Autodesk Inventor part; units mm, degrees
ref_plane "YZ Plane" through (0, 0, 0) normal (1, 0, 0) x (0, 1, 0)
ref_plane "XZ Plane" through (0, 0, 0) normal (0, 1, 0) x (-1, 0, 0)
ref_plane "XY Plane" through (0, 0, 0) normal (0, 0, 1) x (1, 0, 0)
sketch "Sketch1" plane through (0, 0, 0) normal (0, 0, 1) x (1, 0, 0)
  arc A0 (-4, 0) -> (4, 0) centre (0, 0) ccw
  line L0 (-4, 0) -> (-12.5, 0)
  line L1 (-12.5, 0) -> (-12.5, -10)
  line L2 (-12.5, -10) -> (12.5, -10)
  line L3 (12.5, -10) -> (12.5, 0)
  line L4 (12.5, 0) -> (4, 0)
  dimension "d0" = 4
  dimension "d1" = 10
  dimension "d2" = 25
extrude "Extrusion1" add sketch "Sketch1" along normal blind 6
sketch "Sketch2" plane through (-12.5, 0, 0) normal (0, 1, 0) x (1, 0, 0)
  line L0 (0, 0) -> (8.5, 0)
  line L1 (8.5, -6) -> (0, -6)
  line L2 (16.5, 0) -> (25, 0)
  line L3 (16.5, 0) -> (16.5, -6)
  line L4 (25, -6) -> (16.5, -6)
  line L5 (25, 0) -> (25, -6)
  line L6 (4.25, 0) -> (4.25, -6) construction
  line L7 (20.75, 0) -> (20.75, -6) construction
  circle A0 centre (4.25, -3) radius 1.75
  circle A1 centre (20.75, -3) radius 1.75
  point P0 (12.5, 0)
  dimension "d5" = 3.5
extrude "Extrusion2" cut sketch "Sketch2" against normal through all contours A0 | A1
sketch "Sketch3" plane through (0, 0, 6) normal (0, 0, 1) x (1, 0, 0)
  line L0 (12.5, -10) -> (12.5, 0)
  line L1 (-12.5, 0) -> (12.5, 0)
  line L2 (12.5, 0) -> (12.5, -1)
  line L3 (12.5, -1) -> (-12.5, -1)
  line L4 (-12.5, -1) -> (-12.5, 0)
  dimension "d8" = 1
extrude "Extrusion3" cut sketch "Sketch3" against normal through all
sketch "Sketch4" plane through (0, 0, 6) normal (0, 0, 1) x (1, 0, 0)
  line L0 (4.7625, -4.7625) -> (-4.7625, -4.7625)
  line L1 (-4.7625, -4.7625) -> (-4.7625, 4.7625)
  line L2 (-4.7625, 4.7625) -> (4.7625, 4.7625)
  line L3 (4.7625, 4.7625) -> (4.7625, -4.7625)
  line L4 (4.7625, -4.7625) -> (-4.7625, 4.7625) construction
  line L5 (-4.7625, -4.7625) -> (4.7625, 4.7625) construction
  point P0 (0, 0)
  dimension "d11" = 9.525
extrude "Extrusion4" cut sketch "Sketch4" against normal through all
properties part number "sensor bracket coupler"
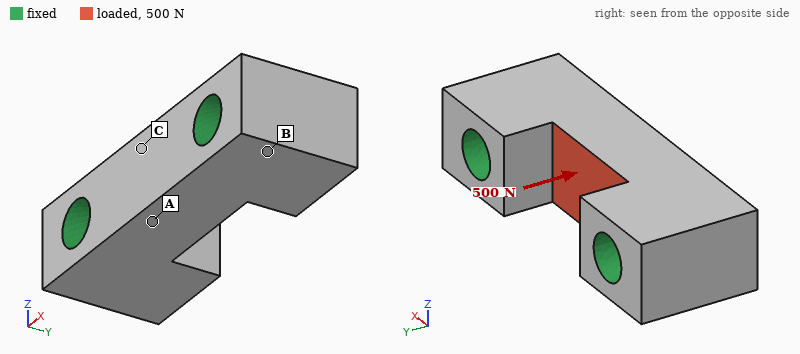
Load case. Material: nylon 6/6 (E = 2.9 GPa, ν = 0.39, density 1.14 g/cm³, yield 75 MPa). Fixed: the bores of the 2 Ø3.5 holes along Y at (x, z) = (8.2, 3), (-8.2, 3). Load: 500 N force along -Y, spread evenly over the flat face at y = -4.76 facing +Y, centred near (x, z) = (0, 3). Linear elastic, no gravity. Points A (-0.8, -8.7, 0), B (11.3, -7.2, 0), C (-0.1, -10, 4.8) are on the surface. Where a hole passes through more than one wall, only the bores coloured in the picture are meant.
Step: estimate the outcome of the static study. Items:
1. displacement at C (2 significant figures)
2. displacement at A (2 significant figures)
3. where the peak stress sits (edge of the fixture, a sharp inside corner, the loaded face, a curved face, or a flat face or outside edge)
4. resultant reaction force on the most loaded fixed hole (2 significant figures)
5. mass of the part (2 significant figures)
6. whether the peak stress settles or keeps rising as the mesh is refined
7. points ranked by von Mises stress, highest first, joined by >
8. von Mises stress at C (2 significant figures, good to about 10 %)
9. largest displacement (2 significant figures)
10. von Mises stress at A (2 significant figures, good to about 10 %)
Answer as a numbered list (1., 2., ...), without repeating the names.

1. 45 µm
2. 48 µm
3. edge of the fixture
4. 250 N
5. 1.1 g
6. keeps rising
7. C > A > B
8. 14 MPa
9. 56 µm
10. 6.8 MPa
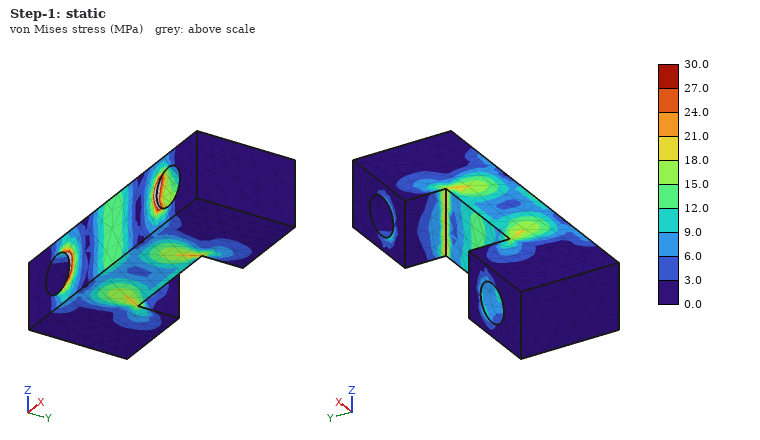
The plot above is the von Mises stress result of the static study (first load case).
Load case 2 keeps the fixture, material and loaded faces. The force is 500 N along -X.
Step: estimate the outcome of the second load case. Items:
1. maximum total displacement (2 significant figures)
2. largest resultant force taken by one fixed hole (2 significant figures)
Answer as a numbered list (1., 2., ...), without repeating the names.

1. 28 µm
2. 260 N
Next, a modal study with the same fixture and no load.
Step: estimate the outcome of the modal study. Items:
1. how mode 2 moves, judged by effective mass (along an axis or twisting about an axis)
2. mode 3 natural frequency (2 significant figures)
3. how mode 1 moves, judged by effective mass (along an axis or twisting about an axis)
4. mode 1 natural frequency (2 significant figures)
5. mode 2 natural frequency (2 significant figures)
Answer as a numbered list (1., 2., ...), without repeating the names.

1. along Y
2. 35 kHz
3. along Z
4. 26 kHz
5. 29 kHz
